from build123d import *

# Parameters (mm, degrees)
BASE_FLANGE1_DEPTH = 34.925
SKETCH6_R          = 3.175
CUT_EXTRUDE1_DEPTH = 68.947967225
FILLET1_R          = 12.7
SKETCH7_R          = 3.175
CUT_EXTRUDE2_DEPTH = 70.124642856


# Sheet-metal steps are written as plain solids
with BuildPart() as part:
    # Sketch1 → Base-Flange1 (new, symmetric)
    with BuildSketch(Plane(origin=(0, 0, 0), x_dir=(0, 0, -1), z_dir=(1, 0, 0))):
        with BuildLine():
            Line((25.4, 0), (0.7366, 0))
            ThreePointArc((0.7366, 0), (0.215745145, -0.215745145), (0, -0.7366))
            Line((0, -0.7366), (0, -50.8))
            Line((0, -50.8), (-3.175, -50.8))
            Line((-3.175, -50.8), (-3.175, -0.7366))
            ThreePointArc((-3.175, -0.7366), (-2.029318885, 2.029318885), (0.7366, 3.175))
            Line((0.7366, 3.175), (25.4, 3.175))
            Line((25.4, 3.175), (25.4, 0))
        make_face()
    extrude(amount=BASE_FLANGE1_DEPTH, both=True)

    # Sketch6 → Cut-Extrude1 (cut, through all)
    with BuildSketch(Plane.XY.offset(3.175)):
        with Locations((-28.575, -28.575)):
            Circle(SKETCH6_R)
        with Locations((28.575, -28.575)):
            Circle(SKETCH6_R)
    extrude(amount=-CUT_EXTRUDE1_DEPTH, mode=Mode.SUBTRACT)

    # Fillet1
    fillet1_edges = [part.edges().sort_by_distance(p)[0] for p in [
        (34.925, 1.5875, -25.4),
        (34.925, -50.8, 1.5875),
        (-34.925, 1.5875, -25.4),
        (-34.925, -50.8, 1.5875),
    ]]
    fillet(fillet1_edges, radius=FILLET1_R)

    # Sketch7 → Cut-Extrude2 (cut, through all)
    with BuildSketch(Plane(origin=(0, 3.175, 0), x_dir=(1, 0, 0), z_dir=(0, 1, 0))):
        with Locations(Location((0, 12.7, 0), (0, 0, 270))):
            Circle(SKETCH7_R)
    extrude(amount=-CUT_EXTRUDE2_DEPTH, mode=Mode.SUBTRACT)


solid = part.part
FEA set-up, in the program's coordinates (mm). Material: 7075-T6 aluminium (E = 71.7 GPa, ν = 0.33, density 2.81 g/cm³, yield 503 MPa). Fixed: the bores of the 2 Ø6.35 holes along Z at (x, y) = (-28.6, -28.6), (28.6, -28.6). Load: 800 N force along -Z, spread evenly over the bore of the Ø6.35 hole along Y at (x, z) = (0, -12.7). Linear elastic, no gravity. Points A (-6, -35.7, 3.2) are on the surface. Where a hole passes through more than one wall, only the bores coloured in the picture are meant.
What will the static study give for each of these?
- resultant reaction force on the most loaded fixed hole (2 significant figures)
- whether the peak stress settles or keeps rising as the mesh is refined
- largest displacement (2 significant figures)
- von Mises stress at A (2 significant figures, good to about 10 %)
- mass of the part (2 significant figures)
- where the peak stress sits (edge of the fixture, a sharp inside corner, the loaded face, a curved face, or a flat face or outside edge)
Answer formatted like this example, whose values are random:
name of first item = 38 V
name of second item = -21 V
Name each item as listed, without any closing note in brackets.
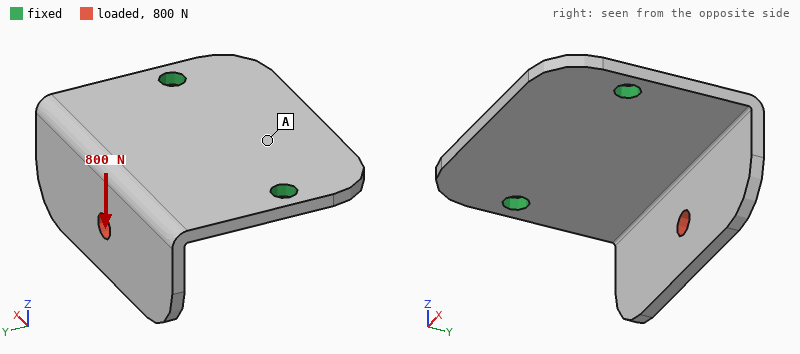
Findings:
resultant reaction force on the most loaded fixed hole = 400 N
whether the peak stress settles or keeps rising as the mesh is refined = keeps rising
largest displacement = 1.00 mm
von Mises stress at A = 33 MPa
mass of the part = 47 g
where the peak stress sits = edge of the fixture
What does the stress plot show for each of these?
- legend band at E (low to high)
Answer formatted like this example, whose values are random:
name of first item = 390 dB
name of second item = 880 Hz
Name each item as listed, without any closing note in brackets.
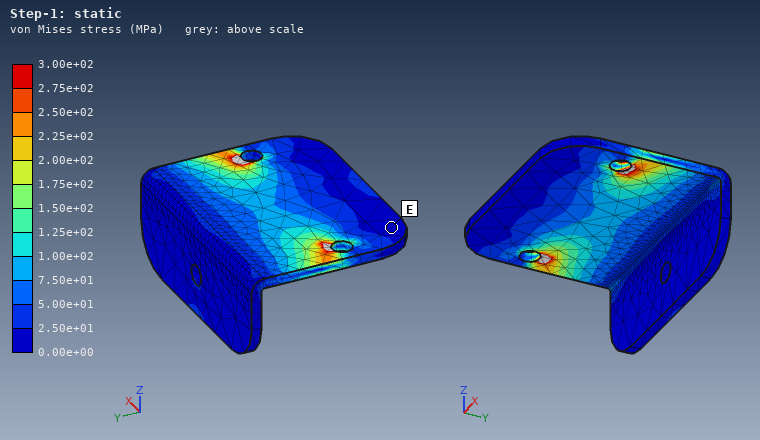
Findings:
legend band at E = 0.00e+00 to 2.50e+01 MPa
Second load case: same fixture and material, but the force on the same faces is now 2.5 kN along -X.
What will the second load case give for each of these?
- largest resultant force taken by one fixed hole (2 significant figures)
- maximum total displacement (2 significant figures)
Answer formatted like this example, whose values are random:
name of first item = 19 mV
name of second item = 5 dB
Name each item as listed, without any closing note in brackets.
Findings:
largest resultant force taken by one fixed hole = 1.9 kN
maximum total displacement = 0.73 mm
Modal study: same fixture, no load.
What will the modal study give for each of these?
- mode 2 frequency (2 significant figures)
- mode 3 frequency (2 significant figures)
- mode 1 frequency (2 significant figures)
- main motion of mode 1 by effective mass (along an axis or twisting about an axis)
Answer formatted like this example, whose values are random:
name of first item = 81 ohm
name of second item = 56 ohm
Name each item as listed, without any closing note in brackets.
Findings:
mode 2 frequency = 2000 Hz
mode 3 frequency = 3000 Hz
mode 1 frequency = 1100 Hz
main motion of mode 1 by effective mass = along Z
